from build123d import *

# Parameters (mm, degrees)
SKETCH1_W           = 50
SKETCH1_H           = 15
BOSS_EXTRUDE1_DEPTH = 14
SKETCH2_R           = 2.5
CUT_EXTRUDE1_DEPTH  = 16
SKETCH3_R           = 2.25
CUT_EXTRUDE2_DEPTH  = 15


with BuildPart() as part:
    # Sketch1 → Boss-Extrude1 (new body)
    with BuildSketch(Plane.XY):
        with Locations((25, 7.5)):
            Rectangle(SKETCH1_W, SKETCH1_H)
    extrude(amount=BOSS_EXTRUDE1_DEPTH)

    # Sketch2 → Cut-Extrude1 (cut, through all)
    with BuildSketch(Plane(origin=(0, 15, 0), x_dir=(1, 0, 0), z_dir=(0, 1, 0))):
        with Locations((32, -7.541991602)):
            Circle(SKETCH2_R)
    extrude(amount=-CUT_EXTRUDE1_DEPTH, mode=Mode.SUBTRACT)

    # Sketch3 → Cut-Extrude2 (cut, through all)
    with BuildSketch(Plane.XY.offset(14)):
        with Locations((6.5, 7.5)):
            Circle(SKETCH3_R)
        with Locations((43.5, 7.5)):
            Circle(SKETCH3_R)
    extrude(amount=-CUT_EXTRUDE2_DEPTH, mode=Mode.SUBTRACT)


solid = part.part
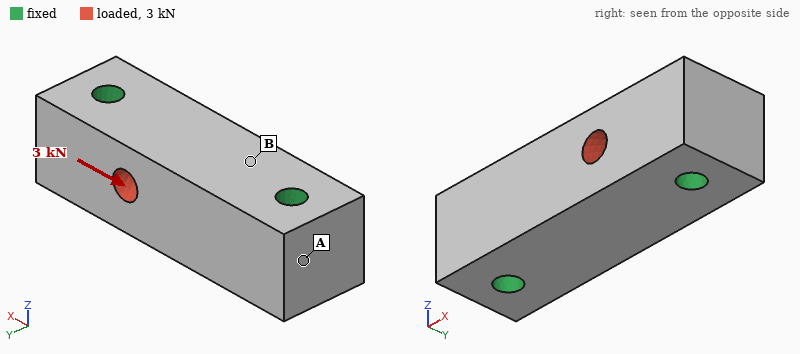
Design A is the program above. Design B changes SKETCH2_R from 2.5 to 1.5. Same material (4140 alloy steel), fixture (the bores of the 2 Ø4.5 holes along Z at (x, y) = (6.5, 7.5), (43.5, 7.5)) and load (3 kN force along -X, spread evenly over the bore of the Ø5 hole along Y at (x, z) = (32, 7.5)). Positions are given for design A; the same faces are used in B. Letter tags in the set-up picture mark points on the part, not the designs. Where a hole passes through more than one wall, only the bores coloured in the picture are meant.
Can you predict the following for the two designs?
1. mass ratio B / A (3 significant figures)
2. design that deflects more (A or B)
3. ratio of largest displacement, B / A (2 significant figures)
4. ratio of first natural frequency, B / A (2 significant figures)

1.02
B
1.1
1.0
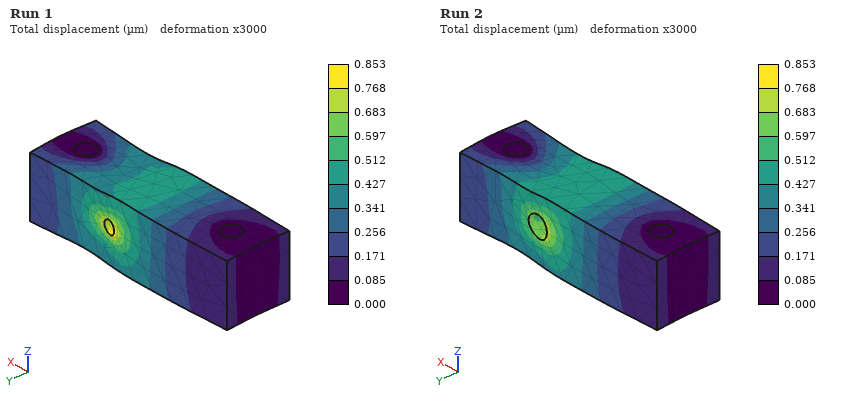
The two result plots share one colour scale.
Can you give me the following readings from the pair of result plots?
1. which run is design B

Run 1
